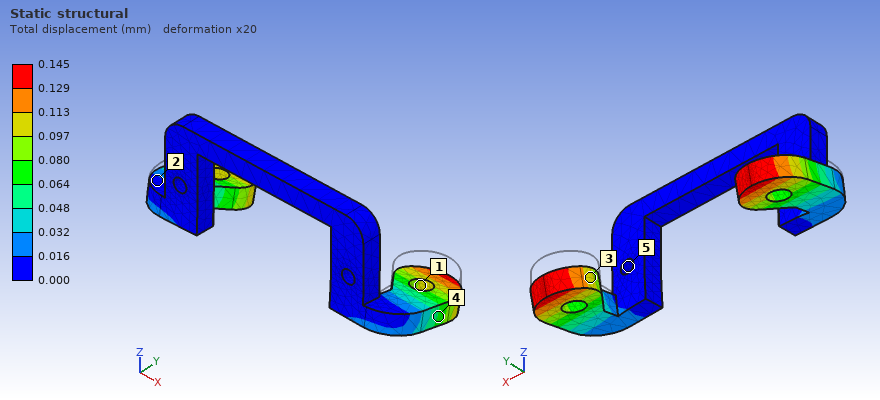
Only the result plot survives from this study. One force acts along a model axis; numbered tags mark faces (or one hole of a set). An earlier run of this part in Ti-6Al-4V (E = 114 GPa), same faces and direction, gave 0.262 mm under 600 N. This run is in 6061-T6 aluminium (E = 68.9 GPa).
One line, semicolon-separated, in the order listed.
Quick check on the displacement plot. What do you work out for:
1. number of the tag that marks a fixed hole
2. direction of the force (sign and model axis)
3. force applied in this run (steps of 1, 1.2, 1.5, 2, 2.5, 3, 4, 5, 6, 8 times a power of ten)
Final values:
5; -Z; 200 N
